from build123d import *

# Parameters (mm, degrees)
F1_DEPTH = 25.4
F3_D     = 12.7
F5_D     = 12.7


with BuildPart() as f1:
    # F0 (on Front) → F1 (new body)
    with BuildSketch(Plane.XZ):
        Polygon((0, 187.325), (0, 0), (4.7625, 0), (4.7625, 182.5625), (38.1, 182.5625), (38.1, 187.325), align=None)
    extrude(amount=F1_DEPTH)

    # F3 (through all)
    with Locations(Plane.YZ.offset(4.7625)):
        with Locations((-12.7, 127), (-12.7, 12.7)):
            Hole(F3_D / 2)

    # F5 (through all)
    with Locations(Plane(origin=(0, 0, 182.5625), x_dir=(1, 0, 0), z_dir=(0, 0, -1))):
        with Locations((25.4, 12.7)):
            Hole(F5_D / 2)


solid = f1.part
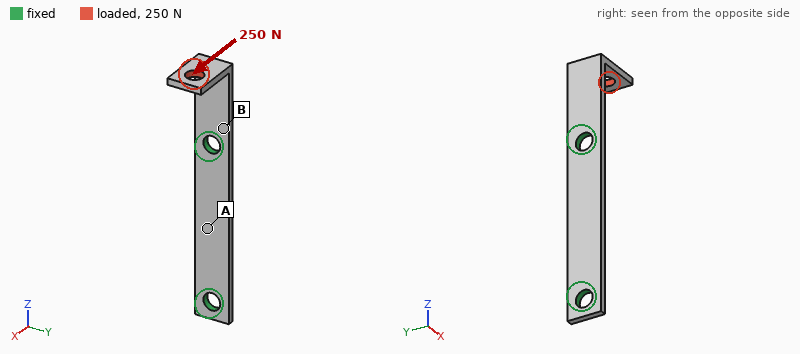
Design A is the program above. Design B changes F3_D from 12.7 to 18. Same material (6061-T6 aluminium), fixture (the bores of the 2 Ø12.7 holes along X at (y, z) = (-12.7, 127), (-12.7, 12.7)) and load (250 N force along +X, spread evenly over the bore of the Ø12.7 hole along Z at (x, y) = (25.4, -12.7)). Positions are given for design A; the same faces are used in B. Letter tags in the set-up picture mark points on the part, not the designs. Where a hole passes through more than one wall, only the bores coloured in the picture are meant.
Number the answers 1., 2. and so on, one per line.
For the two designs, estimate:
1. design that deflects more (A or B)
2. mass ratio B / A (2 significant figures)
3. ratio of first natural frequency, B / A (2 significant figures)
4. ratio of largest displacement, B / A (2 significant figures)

1. A
2. 0.95
3. 1.1
4. 0.87
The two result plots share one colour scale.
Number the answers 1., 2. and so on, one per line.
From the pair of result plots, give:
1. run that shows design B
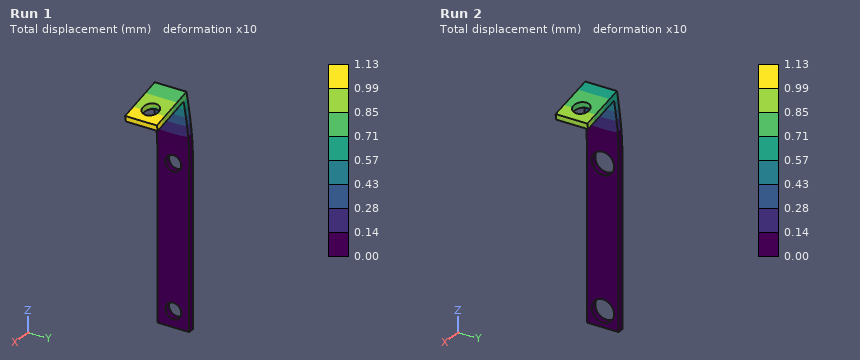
1. Run 2
